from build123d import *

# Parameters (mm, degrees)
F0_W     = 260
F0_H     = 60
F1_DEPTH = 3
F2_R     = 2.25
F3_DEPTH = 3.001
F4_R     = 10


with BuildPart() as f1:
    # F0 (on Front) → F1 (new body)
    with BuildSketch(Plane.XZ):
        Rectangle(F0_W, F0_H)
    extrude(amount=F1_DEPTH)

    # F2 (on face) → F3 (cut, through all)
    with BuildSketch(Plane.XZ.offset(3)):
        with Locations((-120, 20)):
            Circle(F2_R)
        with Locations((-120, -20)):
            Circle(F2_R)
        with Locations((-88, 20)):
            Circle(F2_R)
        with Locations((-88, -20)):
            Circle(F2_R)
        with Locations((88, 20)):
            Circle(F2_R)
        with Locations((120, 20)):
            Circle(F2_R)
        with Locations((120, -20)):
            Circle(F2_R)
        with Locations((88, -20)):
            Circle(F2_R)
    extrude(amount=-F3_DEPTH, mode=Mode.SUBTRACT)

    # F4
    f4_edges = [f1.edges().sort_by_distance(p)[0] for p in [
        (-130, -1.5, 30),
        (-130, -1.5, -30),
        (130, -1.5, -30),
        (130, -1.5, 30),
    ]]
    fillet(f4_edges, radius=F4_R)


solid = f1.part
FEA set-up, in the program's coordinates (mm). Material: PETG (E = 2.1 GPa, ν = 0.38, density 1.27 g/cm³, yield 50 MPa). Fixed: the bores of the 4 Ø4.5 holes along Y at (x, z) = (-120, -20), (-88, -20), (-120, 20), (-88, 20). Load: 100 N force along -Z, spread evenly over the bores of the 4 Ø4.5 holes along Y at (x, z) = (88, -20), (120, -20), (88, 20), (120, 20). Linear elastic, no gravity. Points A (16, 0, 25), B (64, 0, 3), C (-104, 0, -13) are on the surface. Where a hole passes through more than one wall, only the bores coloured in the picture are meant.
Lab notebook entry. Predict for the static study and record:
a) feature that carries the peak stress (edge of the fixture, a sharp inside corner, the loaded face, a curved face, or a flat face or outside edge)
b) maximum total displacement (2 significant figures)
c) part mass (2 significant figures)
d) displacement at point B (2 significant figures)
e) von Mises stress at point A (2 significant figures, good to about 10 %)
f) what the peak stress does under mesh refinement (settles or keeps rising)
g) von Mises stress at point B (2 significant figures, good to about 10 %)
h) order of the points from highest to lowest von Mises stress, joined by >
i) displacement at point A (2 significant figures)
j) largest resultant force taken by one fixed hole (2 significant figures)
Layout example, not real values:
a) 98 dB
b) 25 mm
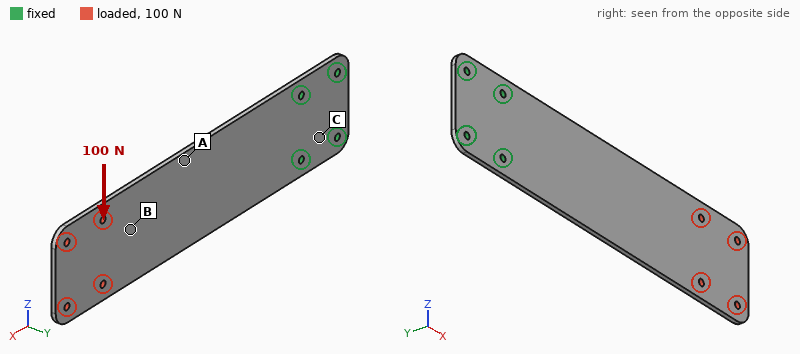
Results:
a) edge of the fixture
b) 2.8 mm
c) 59 g
d) 1.7 mm
e) 4.2 MPa
f) keeps rising
g) 1.4 MPa
h) A > B > C
i) 0.97 mm
j) 390 N
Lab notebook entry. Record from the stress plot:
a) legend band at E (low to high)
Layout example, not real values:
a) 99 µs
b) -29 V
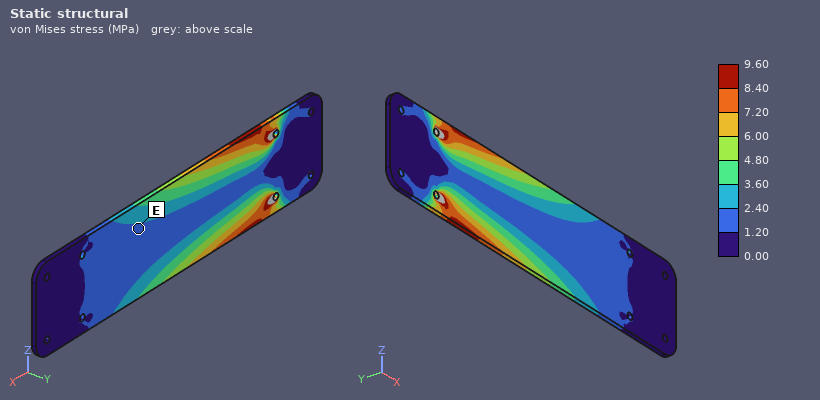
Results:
a) 1.20 to 2.40 MPa
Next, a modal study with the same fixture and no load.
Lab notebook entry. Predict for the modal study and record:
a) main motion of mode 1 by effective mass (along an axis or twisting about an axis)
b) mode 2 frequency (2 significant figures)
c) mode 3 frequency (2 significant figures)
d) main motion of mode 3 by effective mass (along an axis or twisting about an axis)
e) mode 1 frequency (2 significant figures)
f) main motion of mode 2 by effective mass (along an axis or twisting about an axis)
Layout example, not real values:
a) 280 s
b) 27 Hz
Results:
a) along Y
b) 84 Hz
c) 96 Hz
d) twisting about X
e) 13 Hz
f) along Y
